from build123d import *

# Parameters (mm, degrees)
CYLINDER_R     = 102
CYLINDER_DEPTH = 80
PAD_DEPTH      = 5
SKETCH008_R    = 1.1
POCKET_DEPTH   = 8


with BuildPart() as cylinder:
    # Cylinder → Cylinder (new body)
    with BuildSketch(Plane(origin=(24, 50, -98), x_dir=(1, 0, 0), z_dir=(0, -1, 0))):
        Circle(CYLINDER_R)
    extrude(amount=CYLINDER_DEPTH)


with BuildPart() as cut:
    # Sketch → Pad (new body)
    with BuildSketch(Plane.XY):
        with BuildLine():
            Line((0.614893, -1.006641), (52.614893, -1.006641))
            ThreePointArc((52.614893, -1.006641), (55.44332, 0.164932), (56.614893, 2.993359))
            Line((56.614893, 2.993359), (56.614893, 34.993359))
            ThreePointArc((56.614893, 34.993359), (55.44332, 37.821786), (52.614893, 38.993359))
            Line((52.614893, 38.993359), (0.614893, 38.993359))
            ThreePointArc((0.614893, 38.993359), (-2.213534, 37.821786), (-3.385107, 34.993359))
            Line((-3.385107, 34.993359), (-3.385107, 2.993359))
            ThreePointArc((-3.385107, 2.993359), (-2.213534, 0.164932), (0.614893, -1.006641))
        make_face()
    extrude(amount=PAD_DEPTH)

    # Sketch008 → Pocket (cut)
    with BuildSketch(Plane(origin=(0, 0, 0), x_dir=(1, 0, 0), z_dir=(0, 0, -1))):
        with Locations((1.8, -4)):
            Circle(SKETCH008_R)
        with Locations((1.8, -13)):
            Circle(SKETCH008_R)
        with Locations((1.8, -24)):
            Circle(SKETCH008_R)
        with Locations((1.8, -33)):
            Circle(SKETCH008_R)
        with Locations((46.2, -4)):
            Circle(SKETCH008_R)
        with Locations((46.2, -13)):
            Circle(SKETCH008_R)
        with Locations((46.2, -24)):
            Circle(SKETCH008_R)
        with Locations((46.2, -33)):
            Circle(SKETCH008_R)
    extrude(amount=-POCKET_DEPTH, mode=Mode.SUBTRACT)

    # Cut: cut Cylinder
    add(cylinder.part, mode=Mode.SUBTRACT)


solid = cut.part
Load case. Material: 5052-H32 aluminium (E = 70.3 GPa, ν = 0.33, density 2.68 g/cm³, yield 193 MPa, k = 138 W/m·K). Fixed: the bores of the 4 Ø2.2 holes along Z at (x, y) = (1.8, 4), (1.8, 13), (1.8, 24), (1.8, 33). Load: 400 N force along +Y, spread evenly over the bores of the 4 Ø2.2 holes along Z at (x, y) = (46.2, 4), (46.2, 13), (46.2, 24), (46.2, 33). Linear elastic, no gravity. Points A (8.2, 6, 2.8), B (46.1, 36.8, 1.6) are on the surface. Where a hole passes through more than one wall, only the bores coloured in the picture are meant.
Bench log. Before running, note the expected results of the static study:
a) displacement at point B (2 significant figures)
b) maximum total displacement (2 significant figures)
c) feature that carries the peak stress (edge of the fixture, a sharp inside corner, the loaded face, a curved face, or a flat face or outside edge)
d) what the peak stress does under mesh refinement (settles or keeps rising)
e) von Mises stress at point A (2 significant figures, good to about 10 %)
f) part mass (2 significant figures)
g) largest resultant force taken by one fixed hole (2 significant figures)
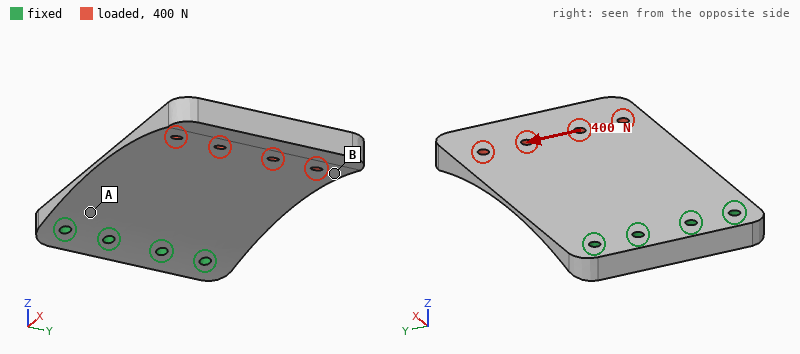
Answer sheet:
0.18 mm
0.21 mm
edge of the fixture
keeps rising
23 MPa
15 g
570 N
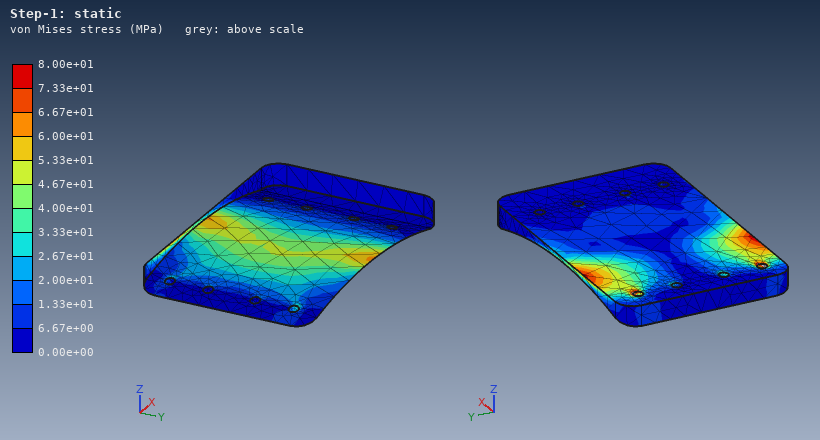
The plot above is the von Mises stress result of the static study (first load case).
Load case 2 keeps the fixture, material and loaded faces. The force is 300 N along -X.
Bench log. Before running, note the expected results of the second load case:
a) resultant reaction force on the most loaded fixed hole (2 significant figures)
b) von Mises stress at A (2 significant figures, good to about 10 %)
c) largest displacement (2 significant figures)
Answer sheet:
85 N
9.2 MPa
0.71 mm
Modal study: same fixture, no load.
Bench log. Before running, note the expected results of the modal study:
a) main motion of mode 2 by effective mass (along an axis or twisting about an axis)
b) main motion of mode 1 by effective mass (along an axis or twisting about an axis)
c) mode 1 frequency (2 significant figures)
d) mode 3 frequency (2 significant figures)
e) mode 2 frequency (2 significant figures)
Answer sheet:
twisting about X
along Z
270 Hz
2900 Hz
1100 Hz
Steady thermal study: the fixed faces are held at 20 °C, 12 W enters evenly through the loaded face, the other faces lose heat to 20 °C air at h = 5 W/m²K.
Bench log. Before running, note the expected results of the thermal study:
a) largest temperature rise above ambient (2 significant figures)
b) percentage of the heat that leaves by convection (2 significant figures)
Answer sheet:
60 K
7.2 %
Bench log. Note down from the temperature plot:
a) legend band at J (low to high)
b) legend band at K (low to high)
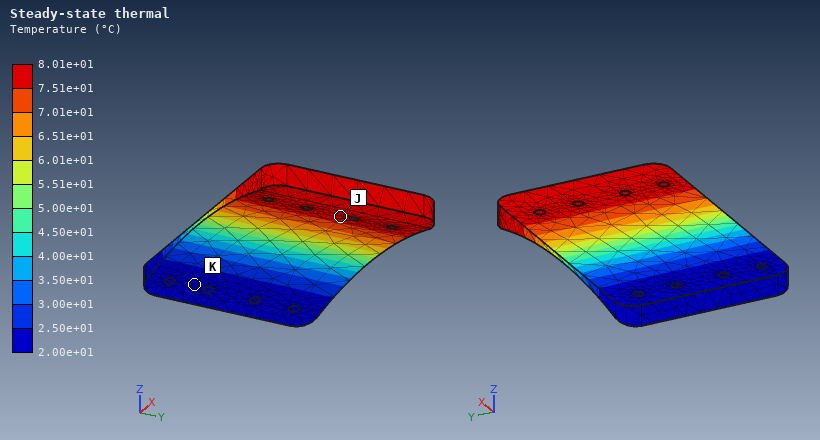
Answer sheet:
7.51e+01 to 8.01e+01 °C
2.00e+01 to 2.50e+01 °C
